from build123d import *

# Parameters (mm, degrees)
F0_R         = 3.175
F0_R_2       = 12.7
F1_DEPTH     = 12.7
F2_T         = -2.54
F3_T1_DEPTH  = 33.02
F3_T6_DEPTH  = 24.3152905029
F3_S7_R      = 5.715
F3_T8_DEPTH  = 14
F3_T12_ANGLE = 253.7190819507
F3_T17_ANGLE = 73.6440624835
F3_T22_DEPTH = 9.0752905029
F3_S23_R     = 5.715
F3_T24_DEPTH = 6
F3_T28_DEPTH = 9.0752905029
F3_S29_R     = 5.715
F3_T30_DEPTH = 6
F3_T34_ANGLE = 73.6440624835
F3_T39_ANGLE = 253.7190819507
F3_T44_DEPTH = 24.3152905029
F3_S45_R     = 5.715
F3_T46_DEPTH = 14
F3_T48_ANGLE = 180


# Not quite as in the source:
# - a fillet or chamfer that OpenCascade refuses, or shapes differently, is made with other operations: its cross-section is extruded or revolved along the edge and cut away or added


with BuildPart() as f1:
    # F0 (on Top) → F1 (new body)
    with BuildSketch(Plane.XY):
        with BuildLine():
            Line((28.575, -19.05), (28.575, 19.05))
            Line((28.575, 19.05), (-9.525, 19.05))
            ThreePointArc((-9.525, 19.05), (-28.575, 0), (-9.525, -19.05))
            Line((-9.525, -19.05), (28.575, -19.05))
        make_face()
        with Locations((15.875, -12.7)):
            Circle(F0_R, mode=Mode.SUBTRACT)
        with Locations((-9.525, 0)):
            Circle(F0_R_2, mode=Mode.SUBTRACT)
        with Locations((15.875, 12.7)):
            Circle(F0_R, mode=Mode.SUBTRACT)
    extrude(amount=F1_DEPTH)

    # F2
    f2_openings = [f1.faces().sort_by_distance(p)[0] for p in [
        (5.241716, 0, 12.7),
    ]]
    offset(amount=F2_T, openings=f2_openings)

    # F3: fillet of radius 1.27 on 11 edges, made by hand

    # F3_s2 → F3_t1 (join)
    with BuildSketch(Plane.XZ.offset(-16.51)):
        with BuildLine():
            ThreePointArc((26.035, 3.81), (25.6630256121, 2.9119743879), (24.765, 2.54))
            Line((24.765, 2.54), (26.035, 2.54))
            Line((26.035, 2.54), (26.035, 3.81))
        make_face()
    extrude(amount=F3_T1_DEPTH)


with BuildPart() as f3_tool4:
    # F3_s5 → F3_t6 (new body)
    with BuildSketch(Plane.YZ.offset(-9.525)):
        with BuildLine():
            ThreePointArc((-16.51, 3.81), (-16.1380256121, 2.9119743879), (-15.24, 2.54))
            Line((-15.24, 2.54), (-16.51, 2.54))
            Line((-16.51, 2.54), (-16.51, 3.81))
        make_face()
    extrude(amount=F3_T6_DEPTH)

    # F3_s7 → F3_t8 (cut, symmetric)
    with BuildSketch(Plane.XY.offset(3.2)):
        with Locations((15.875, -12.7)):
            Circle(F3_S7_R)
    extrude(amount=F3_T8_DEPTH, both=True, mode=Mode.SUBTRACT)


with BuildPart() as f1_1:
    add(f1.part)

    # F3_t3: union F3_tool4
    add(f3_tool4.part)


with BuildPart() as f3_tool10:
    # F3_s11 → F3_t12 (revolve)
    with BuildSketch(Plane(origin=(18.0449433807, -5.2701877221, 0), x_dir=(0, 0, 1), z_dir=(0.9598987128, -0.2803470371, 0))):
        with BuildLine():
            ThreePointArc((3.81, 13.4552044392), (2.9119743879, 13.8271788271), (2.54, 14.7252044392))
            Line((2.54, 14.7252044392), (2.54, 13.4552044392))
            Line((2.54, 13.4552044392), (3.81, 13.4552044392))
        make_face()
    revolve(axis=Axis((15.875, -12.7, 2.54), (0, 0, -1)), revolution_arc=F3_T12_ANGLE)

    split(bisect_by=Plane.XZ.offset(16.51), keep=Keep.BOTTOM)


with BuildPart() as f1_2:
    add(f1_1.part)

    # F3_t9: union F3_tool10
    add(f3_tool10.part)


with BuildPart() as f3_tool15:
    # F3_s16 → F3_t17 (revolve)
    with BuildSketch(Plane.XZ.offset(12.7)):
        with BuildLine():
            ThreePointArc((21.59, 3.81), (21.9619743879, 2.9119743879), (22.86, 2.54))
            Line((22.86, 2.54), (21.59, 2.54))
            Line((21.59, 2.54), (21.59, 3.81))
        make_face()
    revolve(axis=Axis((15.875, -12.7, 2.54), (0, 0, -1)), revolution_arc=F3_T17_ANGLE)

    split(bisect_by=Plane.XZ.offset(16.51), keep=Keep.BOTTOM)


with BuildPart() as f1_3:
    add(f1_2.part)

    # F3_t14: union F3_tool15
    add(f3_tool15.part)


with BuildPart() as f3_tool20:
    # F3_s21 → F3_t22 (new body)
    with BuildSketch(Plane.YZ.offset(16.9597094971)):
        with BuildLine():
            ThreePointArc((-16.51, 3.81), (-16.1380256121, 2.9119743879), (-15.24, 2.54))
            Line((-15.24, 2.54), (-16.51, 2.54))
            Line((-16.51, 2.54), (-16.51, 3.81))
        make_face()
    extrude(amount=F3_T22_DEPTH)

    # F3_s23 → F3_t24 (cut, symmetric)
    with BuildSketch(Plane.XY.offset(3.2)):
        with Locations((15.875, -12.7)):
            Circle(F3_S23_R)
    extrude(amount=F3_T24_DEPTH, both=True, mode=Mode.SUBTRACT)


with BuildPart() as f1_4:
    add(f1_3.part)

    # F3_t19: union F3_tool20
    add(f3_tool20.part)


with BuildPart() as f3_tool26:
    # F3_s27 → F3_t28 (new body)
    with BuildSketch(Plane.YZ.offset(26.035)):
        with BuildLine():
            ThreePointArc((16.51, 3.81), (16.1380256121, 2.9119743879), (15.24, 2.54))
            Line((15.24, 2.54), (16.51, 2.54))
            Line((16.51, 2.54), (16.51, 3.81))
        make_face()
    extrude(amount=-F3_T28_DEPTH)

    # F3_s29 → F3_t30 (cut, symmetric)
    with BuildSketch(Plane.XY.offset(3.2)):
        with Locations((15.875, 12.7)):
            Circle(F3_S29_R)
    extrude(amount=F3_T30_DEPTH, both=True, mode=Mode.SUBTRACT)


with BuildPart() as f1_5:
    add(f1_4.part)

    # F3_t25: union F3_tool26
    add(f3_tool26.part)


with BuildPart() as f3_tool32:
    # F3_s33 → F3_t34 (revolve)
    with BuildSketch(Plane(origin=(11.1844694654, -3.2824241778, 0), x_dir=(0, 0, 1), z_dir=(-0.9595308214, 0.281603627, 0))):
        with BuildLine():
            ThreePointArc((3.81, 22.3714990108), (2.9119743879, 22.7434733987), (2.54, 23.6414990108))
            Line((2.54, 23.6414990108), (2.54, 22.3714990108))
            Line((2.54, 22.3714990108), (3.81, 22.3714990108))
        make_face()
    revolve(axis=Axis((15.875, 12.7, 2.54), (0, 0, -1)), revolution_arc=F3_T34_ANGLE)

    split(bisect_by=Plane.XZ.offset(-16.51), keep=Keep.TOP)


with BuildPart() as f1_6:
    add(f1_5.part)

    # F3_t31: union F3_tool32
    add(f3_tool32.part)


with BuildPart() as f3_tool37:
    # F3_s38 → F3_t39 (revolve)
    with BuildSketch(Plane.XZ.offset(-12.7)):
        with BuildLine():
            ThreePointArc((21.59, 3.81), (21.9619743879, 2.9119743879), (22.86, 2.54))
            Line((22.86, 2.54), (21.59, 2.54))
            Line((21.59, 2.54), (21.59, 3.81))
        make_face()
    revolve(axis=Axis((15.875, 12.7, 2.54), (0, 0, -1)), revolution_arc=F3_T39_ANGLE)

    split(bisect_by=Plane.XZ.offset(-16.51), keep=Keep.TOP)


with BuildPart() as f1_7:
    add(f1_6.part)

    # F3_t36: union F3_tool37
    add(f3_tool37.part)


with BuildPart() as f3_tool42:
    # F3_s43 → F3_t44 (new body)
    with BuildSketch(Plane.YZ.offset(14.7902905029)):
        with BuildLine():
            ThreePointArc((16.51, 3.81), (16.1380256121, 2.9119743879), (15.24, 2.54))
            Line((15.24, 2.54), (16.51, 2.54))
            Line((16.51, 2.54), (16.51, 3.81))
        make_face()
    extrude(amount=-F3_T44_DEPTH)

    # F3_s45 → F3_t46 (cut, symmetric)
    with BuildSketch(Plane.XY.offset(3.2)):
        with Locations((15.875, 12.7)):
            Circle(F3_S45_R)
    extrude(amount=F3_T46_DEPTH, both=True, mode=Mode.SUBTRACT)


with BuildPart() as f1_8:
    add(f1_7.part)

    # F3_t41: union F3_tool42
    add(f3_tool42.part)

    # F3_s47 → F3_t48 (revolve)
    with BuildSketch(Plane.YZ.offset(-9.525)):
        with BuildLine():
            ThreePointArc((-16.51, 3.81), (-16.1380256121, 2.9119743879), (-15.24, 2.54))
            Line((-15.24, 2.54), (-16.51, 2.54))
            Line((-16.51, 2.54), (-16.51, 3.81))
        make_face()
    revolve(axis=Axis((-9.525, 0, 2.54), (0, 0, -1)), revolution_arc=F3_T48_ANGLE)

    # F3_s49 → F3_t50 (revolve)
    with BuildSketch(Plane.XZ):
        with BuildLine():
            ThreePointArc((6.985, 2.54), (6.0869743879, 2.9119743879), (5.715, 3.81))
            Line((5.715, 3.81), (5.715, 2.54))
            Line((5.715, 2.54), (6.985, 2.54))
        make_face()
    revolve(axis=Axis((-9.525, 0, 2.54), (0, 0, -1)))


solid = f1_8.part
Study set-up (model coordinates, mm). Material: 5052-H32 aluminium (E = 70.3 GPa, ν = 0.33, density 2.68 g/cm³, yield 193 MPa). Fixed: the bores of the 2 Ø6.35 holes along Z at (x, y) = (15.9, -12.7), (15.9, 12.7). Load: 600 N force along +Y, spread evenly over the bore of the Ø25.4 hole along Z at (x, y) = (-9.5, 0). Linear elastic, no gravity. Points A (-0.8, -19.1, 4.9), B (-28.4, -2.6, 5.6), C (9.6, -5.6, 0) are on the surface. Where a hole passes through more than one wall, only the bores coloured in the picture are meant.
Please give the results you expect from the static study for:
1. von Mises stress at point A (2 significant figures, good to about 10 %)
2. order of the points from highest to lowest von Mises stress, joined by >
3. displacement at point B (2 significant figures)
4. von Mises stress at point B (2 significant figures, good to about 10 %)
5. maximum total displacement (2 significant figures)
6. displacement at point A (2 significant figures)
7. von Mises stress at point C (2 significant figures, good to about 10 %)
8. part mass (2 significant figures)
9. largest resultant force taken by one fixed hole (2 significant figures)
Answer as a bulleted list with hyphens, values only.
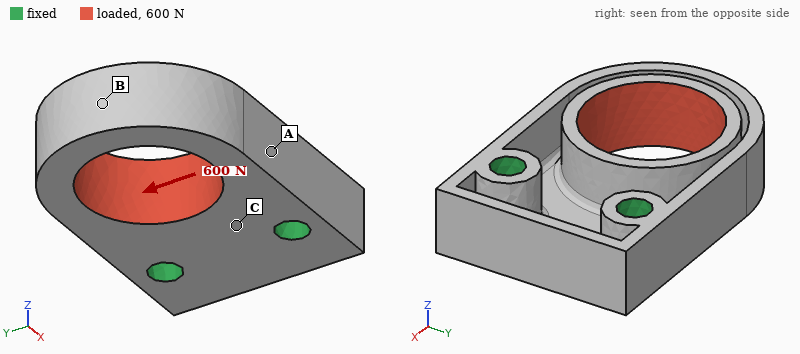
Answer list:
- 18 MPa
- A > C > B
- 32 µm
- 5.5 MPa
- 44 µm
- 11 µm
- 12 MPa
- 31 g
- 540 N
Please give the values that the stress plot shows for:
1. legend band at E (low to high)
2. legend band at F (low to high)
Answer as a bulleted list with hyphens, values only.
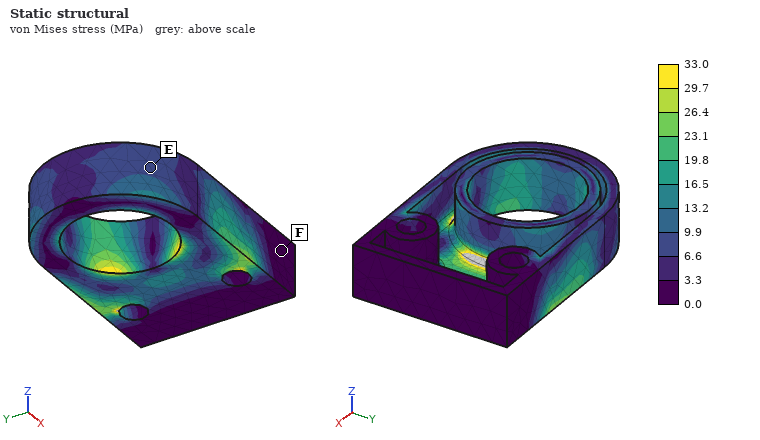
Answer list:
- 6.6 to 9.9 MPa
- 0.0 to 3.3 MPa
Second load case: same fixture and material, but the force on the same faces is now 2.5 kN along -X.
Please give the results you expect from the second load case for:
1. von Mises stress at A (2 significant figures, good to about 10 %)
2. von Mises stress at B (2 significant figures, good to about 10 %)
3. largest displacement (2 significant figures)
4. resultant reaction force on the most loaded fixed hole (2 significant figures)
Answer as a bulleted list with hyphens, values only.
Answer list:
- 23 MPa
- 18 MPa
- 81 µm
- 1.3 kN
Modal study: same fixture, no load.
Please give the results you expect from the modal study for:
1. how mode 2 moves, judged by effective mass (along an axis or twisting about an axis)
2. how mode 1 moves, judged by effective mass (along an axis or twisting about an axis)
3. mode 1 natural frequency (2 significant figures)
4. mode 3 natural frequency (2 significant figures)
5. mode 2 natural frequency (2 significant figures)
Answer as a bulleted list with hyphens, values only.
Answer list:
- along Y
- along Z
- 3700 Hz
- 9300 Hz
- 5100 Hz
